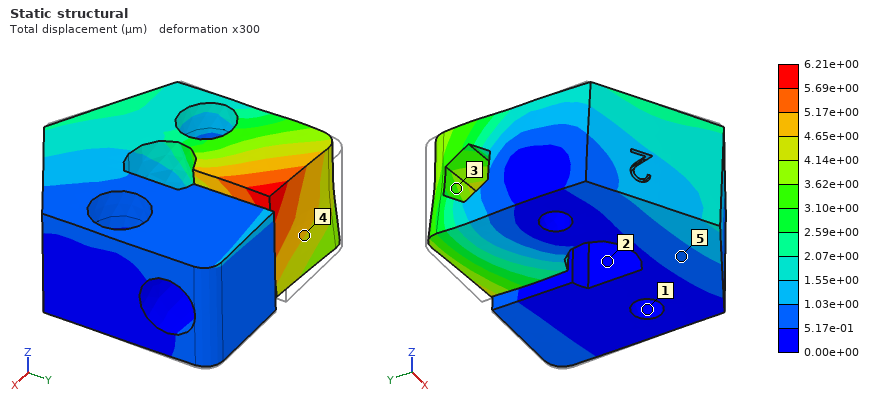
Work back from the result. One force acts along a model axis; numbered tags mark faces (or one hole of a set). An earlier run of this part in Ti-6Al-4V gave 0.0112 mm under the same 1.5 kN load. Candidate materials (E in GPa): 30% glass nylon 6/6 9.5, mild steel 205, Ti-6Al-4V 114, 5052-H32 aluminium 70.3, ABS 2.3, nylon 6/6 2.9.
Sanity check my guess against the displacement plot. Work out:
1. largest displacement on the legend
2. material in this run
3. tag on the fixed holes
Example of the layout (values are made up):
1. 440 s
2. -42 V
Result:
1. 6.21e+00 µm
2. mild steel
3. 1
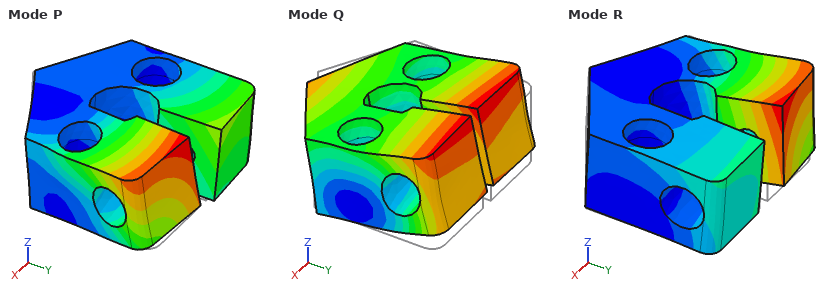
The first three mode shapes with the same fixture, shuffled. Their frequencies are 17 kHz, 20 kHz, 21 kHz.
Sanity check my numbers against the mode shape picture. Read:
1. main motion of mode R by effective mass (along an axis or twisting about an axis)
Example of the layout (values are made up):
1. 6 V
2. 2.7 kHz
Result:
1. along X
